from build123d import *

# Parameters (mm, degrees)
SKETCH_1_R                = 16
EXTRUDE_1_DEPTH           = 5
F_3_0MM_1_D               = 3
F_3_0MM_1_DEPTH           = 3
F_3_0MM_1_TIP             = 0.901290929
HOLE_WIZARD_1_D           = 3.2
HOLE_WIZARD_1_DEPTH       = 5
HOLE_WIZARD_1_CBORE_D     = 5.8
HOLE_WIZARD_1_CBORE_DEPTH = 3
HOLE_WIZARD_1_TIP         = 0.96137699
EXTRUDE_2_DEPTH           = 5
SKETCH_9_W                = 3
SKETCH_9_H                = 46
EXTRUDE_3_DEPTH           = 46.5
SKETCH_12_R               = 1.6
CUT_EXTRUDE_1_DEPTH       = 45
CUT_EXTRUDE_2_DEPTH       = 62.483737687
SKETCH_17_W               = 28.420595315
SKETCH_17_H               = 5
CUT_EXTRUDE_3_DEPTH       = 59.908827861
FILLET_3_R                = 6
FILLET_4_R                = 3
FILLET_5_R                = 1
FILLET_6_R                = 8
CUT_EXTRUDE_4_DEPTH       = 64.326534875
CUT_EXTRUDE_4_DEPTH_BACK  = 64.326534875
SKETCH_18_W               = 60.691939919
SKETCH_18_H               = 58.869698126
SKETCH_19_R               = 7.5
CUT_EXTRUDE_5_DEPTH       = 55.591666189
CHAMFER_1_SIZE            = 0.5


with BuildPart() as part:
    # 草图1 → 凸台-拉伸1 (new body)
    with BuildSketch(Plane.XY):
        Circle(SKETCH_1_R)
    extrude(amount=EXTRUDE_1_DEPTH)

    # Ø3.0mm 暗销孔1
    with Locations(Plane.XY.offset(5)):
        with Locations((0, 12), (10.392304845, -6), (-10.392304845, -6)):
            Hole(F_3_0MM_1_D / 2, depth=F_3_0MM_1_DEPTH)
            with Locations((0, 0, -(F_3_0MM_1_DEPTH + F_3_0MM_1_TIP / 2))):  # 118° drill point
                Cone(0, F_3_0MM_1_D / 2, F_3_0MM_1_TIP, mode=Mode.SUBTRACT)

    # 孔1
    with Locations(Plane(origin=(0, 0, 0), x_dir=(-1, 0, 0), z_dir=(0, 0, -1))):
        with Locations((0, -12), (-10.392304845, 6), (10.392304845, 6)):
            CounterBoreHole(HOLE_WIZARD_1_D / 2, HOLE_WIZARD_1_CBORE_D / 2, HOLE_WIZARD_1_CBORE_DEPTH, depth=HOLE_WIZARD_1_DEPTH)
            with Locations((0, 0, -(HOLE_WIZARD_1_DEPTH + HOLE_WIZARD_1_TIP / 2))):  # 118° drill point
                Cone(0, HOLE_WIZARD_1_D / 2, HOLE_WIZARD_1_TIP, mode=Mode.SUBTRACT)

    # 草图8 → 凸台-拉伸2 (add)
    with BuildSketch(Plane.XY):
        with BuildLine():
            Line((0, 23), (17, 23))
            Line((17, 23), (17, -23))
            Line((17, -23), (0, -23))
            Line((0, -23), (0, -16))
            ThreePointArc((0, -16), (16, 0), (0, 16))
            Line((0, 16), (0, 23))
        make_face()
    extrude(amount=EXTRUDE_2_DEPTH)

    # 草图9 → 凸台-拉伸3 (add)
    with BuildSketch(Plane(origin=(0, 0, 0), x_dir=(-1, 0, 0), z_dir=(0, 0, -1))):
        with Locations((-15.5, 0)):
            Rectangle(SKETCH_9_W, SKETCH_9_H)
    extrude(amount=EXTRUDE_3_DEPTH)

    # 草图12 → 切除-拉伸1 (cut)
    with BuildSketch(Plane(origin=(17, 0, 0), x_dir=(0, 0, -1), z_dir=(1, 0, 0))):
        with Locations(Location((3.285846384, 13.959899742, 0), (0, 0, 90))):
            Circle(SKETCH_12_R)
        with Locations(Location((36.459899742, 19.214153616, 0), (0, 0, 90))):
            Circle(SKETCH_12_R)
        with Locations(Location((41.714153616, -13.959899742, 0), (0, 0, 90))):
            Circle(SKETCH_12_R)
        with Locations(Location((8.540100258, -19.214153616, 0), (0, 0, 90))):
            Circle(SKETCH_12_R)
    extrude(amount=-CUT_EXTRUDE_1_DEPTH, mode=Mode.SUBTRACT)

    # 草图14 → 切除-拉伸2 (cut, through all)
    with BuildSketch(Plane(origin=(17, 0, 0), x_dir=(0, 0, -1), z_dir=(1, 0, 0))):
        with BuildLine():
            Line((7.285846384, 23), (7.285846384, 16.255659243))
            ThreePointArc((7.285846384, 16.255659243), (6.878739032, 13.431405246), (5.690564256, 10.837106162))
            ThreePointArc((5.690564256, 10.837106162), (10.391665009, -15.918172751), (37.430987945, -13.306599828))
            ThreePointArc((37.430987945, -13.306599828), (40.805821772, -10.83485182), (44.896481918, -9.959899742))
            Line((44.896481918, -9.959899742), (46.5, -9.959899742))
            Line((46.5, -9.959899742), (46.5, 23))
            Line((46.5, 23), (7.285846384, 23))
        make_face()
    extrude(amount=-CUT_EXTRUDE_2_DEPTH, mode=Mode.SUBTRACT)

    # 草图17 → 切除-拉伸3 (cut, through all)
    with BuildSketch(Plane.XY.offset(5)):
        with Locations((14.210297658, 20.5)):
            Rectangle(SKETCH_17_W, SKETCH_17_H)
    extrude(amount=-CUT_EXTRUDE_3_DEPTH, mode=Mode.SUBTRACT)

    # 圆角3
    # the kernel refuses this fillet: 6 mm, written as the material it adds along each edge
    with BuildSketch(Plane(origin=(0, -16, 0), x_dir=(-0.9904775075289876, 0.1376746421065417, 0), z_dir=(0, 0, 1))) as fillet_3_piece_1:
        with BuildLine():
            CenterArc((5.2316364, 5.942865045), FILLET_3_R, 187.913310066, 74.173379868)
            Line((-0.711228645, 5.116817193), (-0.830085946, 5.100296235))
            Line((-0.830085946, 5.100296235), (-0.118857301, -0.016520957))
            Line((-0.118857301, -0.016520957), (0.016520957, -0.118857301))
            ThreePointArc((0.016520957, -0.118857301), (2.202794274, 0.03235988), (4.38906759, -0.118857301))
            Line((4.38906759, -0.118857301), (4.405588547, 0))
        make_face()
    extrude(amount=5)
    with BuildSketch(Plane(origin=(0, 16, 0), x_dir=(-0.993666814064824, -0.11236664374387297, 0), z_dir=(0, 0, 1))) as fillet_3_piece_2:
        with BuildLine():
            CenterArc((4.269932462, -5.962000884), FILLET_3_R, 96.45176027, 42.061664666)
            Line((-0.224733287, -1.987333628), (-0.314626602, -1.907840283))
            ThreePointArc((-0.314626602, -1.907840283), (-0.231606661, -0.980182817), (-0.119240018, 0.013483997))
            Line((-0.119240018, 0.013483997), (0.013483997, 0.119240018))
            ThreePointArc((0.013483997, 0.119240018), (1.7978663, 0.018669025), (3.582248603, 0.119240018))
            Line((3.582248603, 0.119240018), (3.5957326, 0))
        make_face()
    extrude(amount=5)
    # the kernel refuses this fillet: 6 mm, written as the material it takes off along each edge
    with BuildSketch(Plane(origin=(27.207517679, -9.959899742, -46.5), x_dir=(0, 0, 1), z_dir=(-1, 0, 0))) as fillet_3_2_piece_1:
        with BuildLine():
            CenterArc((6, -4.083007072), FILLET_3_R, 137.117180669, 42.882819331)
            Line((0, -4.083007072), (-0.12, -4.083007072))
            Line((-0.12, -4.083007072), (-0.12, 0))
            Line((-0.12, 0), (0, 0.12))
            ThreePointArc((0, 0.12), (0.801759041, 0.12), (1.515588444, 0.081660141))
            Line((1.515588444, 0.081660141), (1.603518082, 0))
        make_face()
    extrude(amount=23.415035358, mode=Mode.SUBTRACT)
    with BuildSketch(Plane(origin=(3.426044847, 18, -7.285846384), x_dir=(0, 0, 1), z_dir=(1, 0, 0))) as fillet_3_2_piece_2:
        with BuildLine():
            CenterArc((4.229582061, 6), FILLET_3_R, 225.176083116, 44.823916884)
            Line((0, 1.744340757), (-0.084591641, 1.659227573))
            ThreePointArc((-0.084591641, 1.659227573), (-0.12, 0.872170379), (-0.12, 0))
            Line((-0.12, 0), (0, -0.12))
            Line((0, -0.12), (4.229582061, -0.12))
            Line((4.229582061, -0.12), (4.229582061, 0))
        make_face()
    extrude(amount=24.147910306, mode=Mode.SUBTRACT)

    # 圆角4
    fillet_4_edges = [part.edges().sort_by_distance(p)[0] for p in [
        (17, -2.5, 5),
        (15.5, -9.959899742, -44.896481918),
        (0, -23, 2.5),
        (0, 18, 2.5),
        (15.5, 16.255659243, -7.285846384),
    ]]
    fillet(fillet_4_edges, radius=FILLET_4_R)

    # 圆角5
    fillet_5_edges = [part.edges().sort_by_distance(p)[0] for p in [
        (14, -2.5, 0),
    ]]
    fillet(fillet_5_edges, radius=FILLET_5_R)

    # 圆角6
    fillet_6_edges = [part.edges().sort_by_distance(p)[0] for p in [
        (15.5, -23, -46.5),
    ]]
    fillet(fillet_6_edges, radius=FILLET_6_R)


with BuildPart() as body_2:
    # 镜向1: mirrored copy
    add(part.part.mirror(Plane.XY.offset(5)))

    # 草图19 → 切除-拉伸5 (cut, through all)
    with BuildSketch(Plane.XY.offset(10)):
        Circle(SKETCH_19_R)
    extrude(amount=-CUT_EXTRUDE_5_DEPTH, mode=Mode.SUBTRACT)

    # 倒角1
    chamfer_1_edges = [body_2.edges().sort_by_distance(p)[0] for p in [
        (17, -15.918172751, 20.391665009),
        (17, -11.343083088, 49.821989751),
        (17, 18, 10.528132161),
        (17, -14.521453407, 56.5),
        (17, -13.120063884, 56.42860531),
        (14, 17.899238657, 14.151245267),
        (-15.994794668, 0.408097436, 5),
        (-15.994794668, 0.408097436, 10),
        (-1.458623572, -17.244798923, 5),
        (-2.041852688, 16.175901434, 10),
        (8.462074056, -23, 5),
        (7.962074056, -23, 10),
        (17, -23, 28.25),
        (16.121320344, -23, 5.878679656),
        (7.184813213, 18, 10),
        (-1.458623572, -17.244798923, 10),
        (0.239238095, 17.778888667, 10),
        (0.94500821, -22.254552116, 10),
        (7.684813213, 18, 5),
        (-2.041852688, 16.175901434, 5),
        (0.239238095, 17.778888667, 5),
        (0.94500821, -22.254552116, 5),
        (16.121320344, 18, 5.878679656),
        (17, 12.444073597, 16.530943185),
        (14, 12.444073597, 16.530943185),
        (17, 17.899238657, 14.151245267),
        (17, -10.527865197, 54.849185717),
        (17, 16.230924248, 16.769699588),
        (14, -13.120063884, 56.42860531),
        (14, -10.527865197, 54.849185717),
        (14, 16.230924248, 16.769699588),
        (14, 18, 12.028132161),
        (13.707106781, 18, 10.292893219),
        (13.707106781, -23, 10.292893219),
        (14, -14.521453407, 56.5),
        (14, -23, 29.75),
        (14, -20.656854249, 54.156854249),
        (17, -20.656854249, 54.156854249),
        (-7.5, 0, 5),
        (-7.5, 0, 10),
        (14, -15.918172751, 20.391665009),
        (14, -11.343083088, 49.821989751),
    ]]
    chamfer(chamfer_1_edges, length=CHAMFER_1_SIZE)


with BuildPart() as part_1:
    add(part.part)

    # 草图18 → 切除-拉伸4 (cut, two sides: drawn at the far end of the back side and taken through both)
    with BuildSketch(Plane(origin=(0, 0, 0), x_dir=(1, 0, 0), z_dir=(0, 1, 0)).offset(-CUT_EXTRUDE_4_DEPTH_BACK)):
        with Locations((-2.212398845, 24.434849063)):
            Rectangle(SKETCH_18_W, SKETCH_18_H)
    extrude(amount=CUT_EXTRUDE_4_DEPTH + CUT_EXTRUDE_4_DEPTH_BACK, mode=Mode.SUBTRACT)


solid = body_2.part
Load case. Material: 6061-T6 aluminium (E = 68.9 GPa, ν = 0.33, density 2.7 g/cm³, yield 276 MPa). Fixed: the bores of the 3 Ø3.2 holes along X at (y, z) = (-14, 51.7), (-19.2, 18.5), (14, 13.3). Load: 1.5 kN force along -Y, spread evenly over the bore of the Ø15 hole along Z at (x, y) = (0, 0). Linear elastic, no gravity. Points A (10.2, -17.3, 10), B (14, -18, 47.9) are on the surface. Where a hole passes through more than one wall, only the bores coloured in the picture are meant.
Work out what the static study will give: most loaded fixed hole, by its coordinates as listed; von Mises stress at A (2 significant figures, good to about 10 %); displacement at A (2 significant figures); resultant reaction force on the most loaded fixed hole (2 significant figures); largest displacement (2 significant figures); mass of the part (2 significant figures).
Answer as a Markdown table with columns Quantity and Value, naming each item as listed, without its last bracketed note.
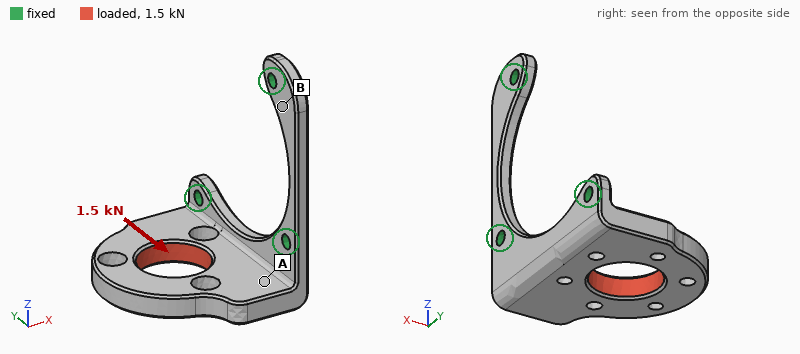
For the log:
| Quantity | Value |
|---|---|
| most loaded fixed hole, by its coordinates as listed | (14, 13.3) |
| von Mises stress at A | 51 MPa |
| displacement at A | 0.072 mm |
| resultant reaction force on the most loaded fixed hole | 1.2 kN |
| largest displacement | 0.18 mm |
| mass of the part | 15 g |
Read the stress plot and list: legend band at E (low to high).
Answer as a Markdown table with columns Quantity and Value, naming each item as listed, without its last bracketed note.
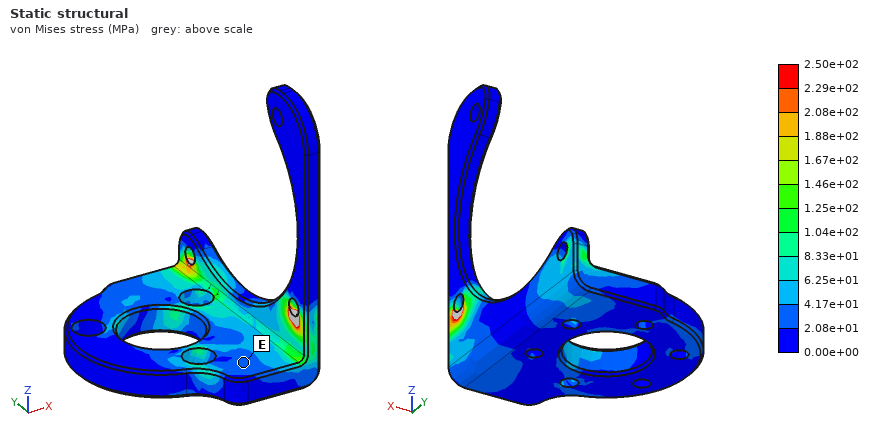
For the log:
| Quantity | Value |
|---|---|
| legend band at E | 2.08e+01 to 4.17e+01 MPa |
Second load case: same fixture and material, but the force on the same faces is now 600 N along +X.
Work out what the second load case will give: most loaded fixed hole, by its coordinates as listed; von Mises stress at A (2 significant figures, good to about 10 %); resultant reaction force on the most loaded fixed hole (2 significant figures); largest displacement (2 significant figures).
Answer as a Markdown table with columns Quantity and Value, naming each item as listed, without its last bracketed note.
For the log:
| Quantity | Value |
|---|---|
| most loaded fixed hole, by its coordinates as listed | (14, 13.3) |
| von Mises stress at A | 13 MPa |
| resultant reaction force on the most loaded fixed hole | 370 N |
| largest displacement | 0.15 mm |
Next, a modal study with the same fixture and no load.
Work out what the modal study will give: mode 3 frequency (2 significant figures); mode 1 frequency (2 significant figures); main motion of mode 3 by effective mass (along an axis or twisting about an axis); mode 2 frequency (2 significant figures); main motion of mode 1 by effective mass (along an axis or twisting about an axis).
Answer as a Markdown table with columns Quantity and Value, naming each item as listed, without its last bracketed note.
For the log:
| Quantity | Value |
|---|---|
| mode 3 frequency | 9800 Hz |
| mode 1 frequency | 2200 Hz |
| main motion of mode 3 by effective mass | along X |
| mode 2 frequency | 6200 Hz |
| main motion of mode 1 by effective mass | along Z |
